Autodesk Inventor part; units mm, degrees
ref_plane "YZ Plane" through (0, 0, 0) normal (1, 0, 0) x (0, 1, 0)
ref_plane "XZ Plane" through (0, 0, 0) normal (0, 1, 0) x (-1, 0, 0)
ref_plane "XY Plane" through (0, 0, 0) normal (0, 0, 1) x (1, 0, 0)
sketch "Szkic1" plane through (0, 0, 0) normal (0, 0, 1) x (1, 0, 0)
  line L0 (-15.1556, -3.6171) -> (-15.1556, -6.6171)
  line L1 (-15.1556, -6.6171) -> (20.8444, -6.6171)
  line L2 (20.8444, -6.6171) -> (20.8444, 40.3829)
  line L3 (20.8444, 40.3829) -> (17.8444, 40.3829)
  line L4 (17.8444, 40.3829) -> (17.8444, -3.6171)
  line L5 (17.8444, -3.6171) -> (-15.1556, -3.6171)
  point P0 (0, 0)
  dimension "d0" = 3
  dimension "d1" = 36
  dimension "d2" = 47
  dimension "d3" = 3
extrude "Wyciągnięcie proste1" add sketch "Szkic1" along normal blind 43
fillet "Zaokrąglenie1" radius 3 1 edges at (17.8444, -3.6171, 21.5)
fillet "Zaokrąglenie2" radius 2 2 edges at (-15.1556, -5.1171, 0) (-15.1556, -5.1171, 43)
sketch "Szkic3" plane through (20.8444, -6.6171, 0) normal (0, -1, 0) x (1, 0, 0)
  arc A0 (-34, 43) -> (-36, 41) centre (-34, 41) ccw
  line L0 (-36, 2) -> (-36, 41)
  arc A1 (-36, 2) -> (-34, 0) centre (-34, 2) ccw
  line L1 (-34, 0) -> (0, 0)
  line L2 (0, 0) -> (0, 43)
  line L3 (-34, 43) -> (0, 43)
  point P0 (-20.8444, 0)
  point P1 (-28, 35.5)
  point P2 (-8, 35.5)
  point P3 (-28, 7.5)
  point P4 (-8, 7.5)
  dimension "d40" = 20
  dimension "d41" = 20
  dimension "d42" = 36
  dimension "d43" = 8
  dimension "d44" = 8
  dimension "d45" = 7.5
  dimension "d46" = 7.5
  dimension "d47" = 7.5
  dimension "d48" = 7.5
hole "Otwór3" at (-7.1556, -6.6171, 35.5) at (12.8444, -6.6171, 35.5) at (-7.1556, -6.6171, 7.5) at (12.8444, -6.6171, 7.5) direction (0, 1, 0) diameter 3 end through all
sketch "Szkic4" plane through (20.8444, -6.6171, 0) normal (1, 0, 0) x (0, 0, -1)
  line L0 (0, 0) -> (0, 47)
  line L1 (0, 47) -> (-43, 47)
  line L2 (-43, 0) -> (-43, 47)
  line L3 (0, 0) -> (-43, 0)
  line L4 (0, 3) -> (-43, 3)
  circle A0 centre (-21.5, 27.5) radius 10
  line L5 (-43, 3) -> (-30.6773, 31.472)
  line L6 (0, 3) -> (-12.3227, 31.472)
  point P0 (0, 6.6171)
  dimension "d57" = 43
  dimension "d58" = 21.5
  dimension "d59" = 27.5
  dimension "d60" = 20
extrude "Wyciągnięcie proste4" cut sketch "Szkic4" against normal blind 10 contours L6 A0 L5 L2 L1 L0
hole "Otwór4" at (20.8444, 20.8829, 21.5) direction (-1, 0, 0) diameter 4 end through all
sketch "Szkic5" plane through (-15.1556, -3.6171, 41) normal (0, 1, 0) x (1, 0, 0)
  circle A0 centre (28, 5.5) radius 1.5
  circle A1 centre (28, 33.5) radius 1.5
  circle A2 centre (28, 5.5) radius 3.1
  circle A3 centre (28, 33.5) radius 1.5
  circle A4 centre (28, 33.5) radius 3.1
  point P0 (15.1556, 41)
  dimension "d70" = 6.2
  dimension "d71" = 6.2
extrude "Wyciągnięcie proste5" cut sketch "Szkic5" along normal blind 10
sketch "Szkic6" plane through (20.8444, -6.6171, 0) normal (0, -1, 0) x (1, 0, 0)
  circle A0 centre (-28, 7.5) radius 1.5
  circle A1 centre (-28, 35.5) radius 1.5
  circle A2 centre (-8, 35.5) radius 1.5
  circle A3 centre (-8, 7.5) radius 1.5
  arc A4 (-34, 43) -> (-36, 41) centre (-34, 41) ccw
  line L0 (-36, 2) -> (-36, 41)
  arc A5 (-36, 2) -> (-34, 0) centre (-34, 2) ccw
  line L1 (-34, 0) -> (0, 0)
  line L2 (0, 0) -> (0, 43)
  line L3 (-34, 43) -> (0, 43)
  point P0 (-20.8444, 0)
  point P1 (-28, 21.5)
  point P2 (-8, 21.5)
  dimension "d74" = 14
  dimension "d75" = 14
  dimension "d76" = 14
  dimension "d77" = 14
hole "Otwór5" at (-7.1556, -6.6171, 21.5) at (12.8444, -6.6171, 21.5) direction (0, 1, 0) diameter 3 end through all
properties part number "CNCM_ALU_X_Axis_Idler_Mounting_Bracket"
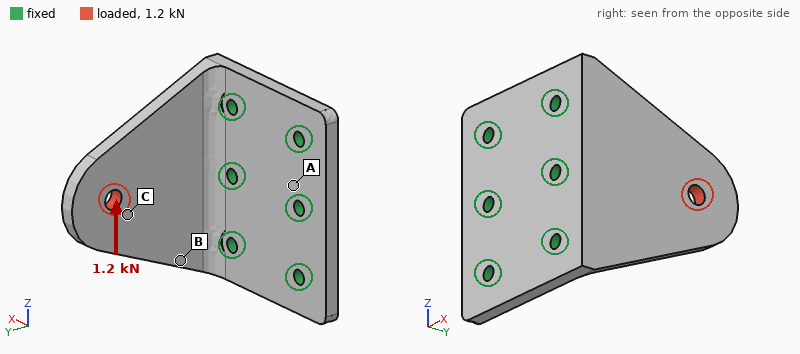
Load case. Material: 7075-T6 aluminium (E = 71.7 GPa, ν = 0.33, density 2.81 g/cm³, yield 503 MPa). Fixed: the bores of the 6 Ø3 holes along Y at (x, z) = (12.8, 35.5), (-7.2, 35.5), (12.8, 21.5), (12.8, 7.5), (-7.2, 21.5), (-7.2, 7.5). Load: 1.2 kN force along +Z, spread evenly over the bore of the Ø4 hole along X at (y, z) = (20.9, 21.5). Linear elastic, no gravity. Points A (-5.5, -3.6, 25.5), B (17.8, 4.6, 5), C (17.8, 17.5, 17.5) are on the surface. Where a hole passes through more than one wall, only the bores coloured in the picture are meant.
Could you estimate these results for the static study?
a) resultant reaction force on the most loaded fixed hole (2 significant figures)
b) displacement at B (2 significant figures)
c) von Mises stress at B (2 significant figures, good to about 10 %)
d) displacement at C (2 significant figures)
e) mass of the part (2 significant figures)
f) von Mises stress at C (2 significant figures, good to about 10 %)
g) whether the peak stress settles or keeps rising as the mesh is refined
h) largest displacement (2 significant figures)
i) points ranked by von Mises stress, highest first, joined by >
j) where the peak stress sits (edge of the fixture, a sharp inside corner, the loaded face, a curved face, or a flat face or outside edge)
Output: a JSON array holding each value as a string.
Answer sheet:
["1.2 kN", "56 µm", "70 MPa", "66 µm", "21 g", "37 MPa", "keeps rising", "98 µm", "B > C > A", "edge of the fixture"]
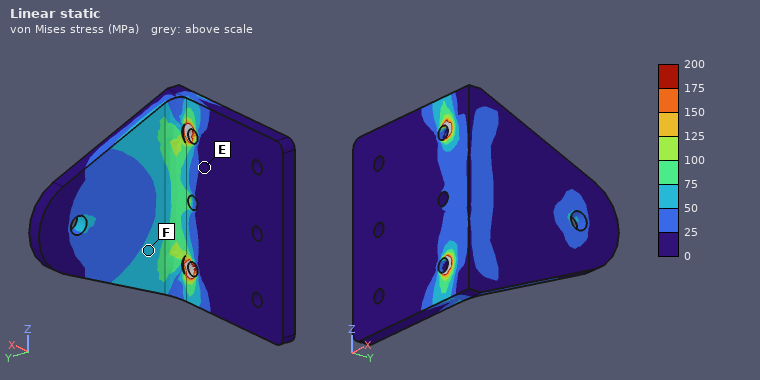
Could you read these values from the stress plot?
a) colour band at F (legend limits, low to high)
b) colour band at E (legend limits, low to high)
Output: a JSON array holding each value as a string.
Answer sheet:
["50 to 75 MPa", "0 to 25 MPa"]
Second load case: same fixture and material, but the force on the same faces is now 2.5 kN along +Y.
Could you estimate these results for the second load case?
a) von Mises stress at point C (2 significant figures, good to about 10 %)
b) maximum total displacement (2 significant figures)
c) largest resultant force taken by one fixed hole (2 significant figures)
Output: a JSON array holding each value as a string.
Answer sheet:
["46 MPa", "0.25 mm", "920 N"]
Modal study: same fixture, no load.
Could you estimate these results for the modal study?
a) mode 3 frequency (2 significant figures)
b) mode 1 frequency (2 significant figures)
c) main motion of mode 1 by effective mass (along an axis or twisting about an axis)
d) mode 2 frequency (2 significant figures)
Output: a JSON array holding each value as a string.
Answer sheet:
["11 kHz", "2500 Hz", "along X", "7700 Hz"]
